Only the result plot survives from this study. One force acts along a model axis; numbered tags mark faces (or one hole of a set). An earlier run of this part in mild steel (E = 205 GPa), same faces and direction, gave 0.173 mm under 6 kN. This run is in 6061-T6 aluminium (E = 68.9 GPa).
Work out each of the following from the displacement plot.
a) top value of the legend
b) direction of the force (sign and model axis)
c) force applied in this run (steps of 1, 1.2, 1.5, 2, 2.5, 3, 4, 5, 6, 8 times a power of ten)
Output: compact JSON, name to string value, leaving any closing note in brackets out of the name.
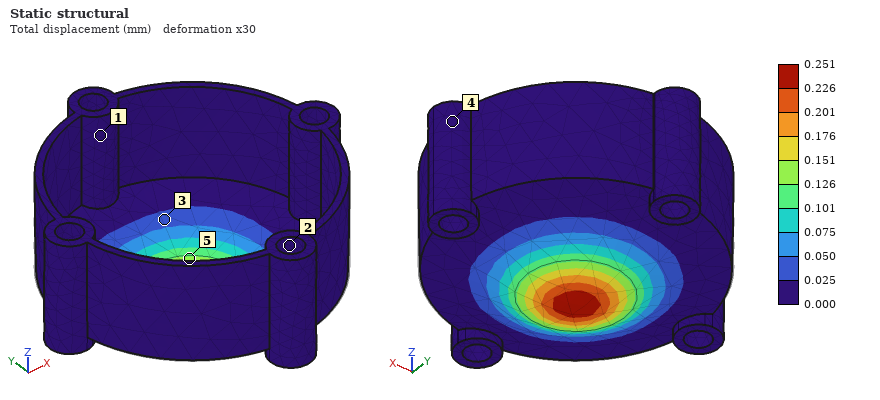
{"top value of the legend": "0.251 mm", "direction of the force": "-Z", "force applied in this run": "3 kN"}
